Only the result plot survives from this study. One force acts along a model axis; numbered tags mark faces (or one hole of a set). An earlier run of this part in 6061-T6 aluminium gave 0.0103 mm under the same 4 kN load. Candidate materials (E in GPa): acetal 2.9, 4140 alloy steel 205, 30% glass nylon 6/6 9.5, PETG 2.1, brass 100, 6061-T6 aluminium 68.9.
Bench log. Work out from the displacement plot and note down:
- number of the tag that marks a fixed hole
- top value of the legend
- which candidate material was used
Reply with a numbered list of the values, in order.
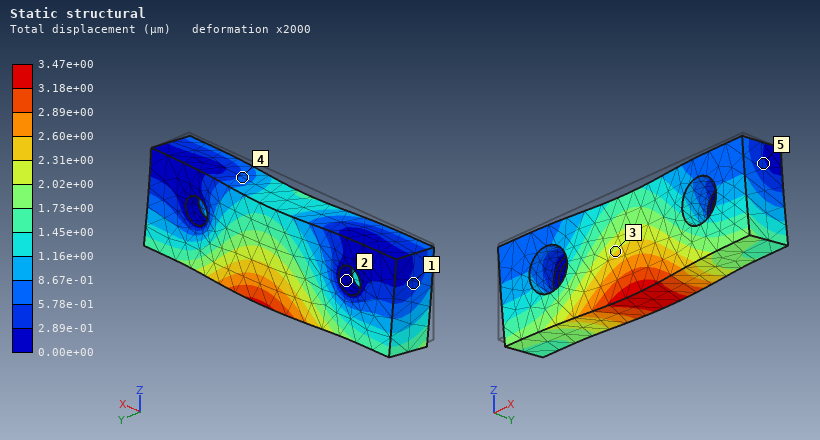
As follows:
1. 2
2. 3.47e+00 µm
3. 4140 alloy steel
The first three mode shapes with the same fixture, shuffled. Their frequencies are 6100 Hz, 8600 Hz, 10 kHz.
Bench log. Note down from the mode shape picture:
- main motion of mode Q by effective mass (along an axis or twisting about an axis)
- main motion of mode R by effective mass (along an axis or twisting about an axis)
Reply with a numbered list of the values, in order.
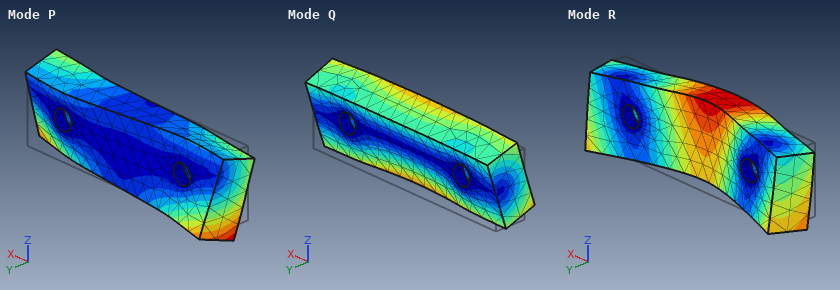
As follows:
1. along Z
2. along Y
